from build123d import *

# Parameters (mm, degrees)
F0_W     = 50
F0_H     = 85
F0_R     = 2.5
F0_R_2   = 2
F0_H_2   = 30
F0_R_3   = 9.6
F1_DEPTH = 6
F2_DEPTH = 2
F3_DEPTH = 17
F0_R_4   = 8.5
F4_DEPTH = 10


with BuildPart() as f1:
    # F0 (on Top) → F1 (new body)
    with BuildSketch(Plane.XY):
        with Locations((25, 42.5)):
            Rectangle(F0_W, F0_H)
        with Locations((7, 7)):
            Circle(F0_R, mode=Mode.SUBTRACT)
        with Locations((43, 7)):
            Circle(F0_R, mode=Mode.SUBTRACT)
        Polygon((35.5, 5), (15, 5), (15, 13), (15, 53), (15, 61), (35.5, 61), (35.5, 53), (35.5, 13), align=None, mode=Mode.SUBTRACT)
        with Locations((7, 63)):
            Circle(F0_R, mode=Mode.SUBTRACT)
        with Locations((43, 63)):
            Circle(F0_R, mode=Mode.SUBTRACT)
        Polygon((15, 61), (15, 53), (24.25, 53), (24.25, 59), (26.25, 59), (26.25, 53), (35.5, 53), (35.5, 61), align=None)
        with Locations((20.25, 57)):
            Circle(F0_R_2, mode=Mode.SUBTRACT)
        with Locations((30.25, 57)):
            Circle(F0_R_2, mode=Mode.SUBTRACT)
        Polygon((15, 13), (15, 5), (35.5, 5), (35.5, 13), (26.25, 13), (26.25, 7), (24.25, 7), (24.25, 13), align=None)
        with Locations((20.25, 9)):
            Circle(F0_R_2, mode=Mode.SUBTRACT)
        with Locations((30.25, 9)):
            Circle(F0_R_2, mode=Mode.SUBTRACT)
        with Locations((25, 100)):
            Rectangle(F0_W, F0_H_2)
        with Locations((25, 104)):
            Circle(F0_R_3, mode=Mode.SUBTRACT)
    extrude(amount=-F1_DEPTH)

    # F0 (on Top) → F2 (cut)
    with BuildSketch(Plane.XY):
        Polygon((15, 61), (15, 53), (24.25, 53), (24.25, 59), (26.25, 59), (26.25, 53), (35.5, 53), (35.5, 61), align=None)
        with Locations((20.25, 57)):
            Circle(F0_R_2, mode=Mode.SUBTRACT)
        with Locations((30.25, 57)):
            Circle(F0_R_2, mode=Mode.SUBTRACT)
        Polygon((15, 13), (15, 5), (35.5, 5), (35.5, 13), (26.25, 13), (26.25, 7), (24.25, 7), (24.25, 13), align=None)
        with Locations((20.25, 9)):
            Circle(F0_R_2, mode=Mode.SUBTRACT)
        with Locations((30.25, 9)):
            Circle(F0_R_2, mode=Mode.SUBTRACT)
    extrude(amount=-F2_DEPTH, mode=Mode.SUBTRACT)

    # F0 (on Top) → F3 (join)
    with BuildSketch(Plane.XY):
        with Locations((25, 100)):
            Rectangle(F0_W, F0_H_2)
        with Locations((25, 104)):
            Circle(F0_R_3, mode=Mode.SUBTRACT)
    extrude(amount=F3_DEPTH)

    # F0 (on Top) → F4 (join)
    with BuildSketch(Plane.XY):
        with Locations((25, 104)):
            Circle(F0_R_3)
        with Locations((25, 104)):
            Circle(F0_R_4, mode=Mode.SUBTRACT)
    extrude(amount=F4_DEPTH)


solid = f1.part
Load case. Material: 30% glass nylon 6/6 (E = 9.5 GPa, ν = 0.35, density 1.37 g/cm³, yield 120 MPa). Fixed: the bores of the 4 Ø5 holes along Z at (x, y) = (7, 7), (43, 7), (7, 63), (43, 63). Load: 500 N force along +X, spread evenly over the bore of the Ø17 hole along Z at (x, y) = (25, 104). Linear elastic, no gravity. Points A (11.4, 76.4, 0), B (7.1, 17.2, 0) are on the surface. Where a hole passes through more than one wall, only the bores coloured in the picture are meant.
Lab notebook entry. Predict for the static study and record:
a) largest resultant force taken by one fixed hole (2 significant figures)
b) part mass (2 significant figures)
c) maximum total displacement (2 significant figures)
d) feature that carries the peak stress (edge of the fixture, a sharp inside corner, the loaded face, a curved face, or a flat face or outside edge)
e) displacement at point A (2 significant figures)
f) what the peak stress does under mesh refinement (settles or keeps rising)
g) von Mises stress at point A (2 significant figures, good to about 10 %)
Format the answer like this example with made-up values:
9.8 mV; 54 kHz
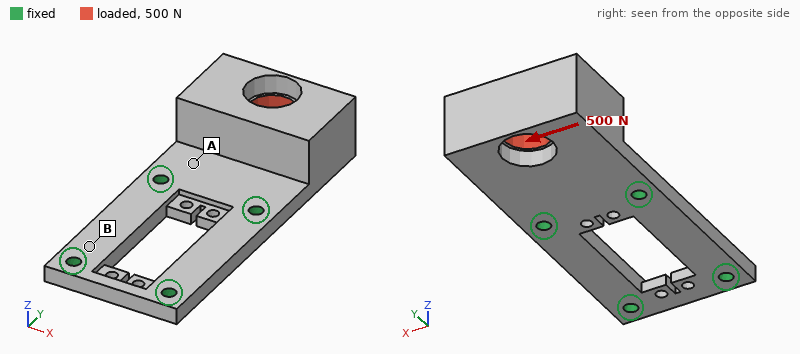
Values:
580 N; 65 g; 0.10 mm; edge of the fixture; 0.021 mm; keeps rising; 8.2 MPa
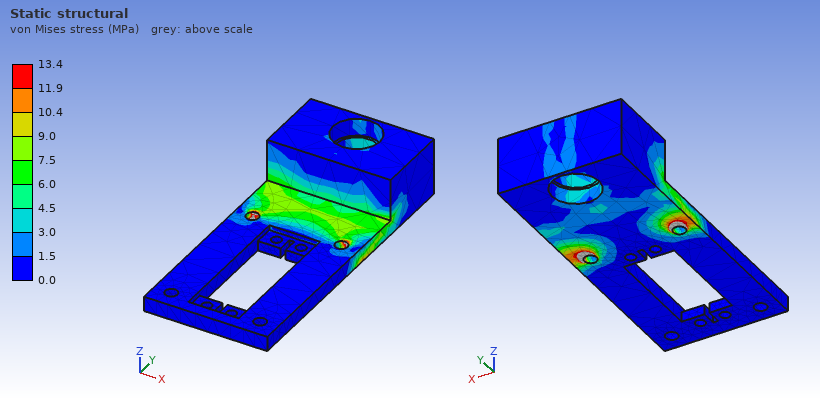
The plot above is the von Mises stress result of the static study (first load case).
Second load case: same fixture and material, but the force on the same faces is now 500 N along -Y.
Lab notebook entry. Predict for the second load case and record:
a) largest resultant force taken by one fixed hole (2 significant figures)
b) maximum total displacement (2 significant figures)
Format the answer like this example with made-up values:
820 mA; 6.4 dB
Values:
250 N; 0.52 mm
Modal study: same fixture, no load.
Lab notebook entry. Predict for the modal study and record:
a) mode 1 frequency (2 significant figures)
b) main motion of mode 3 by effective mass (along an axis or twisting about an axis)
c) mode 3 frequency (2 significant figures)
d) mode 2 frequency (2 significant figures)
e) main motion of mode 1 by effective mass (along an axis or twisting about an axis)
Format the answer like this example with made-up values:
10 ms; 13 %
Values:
510 Hz; along X; 3000 Hz; 1600 Hz; along Z
